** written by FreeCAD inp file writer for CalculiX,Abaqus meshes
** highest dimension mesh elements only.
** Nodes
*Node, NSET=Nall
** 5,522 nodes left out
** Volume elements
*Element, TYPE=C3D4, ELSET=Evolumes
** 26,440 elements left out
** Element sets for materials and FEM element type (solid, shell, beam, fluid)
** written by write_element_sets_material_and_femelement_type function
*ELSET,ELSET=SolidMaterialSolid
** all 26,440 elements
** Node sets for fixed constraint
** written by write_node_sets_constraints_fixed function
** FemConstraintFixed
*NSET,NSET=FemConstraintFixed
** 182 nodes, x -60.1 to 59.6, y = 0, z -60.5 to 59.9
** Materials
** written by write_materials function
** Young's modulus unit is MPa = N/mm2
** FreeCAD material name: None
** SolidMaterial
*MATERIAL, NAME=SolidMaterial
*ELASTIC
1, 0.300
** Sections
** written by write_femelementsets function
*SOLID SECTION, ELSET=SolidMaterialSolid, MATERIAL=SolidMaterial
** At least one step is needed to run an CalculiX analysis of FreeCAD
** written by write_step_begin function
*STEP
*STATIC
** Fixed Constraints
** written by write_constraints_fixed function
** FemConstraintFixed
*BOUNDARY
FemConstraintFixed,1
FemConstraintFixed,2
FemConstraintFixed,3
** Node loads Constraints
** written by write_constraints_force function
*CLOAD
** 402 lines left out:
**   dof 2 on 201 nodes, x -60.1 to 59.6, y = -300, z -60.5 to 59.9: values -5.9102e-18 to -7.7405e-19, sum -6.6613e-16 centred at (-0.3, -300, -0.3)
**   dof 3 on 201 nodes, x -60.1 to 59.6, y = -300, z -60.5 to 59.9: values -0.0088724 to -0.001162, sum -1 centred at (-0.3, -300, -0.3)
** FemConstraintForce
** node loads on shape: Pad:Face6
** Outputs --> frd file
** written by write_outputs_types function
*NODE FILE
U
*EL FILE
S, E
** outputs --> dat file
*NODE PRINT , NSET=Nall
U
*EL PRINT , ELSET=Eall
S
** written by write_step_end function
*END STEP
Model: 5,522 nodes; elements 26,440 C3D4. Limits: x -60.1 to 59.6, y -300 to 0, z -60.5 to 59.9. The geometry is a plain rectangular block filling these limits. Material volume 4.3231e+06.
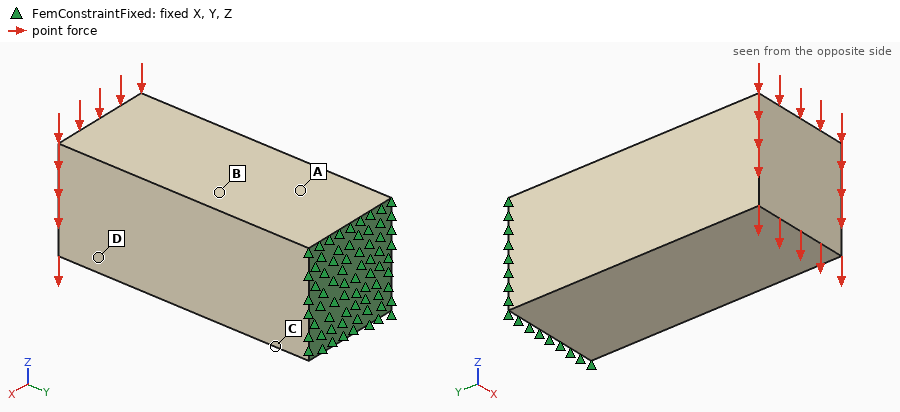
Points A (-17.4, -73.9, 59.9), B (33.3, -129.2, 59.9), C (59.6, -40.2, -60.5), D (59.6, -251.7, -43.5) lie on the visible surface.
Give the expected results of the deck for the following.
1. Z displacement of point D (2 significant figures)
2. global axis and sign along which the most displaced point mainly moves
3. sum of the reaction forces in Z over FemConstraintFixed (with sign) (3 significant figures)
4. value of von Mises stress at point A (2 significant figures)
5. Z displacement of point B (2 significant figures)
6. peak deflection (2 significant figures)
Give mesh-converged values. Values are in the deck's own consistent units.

-0.43
-Z
1.00
7.8e-04
-0.15
0.59
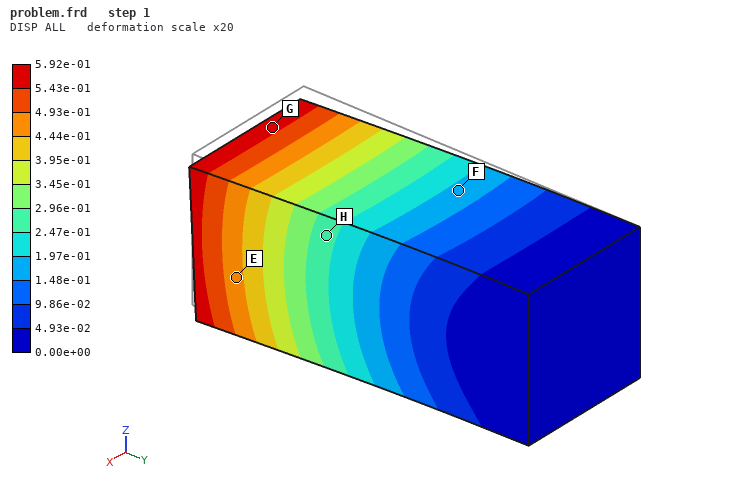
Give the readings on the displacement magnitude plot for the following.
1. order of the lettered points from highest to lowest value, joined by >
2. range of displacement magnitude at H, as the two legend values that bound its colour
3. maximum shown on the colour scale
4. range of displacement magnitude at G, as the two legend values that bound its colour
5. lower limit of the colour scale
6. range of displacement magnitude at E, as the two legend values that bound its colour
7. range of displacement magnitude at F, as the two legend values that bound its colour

G > E > H > F
2.47e-01 to 2.96e-01
5.92e-01
5.43e-01 to 5.92e-01
0.00e+00
4.44e-01 to 4.93e-01
1.48e-01 to 1.97e-01
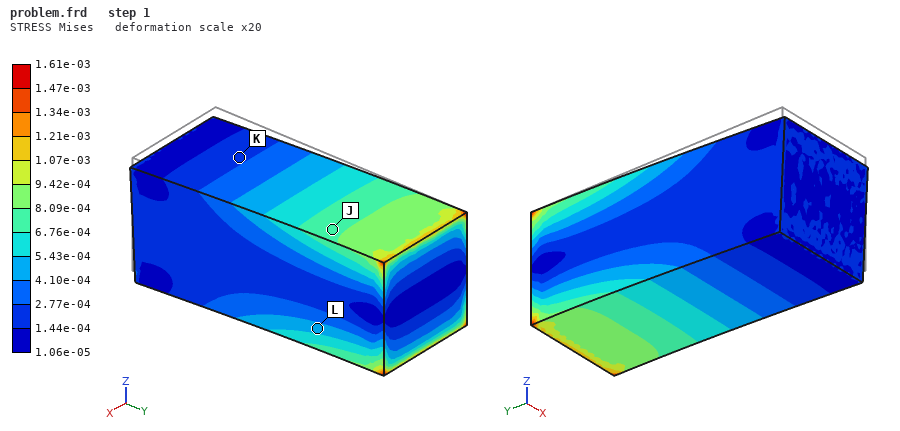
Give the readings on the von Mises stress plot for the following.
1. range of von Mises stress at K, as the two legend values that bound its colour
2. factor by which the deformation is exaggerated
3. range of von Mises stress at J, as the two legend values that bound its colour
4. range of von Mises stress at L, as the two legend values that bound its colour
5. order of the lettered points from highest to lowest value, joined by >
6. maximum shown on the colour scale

1.44e-04 to 2.77e-04
20
6.76e-04 to 8.09e-04
4.10e-04 to 5.43e-04
J > L > K
1.61e-03
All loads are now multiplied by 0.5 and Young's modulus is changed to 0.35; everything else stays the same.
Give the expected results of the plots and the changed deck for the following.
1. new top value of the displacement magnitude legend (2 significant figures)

0.85
